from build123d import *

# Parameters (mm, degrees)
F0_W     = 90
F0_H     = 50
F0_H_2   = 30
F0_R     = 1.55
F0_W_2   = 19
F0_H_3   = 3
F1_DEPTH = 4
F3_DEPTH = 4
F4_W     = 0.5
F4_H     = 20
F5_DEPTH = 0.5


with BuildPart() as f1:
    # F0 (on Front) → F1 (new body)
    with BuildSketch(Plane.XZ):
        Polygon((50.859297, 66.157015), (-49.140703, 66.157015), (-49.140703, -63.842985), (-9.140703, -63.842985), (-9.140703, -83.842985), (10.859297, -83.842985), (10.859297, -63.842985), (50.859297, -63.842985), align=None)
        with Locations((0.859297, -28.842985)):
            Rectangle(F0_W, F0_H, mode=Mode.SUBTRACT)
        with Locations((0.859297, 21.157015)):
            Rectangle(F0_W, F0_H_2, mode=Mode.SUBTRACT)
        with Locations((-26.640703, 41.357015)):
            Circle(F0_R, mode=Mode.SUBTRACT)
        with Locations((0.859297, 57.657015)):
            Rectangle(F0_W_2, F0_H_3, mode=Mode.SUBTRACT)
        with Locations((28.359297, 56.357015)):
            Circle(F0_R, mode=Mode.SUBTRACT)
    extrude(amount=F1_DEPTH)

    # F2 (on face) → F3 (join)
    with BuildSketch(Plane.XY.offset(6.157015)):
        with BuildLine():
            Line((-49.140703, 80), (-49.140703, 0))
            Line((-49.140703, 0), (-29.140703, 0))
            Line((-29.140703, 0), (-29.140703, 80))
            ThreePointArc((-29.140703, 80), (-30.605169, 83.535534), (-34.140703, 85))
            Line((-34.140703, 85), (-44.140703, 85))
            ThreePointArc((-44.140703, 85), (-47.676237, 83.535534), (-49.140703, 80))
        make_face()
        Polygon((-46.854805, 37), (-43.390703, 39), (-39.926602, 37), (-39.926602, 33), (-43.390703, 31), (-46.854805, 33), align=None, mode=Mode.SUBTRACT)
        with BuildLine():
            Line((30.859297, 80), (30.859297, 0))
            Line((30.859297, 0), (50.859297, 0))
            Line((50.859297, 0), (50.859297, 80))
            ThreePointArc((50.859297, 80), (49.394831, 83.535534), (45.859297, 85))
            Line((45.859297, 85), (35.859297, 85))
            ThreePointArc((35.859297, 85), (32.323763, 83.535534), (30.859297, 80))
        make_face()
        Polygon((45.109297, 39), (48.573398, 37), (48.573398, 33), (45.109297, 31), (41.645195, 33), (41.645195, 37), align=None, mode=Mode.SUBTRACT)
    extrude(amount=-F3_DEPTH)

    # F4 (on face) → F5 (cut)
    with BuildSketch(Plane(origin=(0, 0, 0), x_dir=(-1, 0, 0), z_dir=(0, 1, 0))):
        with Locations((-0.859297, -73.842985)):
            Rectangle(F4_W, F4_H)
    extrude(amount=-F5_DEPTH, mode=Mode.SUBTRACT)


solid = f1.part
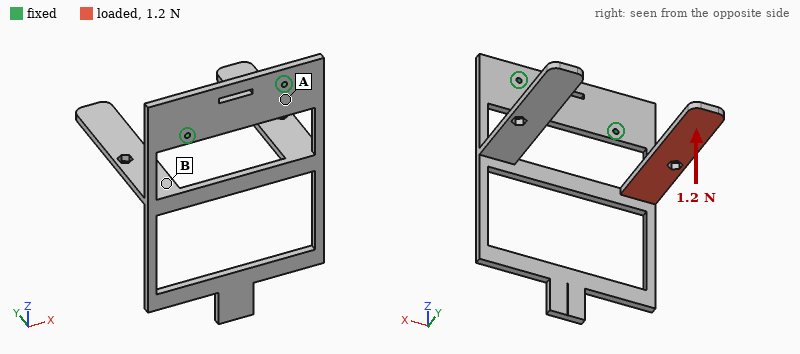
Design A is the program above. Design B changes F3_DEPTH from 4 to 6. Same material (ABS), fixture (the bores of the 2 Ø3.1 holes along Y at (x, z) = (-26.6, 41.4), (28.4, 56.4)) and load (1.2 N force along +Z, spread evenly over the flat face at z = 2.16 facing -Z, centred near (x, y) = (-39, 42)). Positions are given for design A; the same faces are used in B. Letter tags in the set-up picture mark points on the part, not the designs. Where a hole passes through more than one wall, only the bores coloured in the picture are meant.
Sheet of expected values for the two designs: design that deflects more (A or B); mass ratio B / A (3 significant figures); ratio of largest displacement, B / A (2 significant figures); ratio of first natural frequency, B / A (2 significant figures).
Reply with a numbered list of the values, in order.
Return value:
1. A
2. 1.17
3. 0.87
4. 0.92
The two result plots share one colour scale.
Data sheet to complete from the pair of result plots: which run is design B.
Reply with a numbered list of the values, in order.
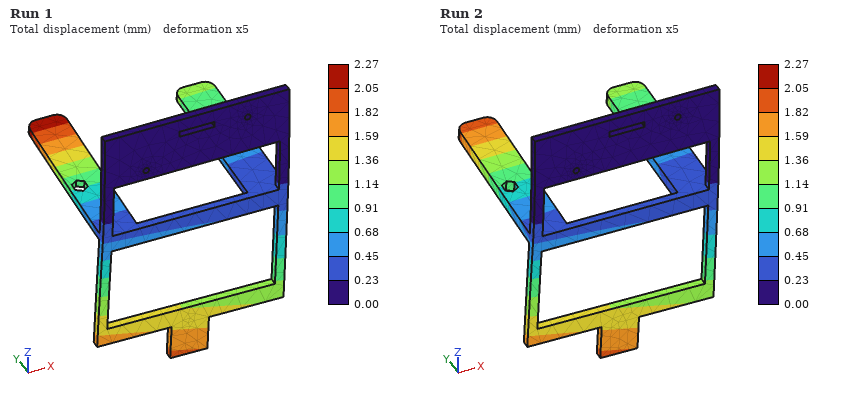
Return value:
1. Run 2
